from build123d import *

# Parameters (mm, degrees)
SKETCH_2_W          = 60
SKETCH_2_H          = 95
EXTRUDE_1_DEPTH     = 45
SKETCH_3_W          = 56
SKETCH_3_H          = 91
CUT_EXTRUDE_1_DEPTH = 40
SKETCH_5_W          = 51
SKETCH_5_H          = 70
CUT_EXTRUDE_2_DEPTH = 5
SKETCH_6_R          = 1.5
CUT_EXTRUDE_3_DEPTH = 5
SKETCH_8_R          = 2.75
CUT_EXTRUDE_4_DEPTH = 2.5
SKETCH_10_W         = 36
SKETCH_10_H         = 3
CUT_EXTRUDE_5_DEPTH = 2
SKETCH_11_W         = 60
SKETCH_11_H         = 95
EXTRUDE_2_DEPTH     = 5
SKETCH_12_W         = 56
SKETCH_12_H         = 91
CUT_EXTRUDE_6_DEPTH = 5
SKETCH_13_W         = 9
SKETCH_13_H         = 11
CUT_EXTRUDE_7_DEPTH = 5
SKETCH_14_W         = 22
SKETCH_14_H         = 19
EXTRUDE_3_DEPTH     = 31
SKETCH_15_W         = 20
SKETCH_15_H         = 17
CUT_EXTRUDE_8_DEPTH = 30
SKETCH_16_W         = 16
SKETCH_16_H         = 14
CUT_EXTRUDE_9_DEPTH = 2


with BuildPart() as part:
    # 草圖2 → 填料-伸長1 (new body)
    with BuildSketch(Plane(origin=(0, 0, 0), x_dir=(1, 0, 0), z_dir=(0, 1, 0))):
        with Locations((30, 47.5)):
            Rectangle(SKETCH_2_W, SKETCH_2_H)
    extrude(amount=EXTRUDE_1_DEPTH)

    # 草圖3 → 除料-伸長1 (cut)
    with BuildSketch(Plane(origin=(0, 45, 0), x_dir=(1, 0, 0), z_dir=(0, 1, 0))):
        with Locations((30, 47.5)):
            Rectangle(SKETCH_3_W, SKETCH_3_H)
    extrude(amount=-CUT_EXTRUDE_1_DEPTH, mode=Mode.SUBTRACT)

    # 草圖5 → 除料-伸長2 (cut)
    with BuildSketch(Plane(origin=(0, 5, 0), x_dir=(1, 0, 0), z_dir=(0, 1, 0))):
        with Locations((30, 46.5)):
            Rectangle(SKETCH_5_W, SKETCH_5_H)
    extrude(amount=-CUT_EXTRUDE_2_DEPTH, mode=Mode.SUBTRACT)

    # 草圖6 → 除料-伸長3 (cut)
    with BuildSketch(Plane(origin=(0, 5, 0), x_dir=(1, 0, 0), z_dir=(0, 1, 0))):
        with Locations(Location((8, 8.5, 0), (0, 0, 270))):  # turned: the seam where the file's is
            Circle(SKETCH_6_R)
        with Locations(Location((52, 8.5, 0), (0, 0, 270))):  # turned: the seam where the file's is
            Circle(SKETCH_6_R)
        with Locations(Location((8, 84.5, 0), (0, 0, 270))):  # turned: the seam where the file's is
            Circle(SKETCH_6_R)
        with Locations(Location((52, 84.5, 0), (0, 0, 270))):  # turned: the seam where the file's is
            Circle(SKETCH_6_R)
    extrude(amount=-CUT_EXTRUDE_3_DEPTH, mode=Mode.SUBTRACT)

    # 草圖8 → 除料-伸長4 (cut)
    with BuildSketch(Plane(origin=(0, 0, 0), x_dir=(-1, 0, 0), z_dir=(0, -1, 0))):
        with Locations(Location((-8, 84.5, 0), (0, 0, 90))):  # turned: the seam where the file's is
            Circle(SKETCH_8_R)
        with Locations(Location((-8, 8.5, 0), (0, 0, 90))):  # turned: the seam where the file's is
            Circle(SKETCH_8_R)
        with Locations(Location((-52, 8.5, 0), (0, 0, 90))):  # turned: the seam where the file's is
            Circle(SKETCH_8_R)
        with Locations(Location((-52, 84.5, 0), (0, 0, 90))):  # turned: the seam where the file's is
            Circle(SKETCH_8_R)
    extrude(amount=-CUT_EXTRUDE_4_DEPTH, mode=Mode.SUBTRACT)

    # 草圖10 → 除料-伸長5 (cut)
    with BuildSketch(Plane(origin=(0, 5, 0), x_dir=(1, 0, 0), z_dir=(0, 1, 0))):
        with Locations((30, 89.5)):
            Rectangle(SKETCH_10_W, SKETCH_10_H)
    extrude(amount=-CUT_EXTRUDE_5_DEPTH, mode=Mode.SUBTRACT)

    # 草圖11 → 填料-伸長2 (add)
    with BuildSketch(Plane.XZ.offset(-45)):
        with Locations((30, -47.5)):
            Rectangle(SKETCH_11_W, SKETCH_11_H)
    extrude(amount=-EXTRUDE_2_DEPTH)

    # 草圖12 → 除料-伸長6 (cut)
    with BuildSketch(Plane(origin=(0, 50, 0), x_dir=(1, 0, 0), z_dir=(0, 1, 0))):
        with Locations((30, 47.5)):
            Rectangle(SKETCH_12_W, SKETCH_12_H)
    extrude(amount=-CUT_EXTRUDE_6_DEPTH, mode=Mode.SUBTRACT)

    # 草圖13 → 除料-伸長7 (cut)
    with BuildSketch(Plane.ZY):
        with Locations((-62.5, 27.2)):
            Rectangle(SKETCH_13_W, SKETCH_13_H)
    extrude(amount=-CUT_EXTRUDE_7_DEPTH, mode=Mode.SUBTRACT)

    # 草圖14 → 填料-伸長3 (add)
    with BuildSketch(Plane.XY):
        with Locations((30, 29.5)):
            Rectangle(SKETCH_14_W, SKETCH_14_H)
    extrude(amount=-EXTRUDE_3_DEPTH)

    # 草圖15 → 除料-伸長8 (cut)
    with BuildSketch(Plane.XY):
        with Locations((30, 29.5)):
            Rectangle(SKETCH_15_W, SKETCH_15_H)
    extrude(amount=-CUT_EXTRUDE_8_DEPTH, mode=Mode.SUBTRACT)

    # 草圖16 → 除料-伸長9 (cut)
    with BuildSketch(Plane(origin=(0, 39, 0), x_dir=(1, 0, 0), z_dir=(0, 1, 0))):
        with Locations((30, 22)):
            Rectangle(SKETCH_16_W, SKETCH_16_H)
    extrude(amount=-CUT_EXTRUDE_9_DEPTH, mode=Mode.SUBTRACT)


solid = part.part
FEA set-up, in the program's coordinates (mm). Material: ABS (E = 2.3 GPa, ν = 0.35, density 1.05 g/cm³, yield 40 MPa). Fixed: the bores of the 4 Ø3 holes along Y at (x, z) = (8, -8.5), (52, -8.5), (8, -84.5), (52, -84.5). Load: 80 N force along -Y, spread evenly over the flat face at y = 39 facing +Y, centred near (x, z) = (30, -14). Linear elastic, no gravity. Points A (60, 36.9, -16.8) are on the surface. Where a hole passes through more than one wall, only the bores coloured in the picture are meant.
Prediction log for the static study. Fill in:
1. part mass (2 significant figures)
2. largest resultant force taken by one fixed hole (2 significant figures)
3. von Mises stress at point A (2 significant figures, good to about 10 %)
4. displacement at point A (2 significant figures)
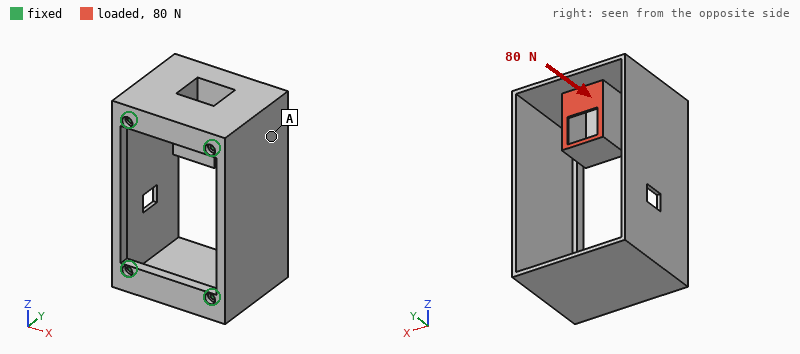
41 g
37 N
1.8 MPa
0.27 mm
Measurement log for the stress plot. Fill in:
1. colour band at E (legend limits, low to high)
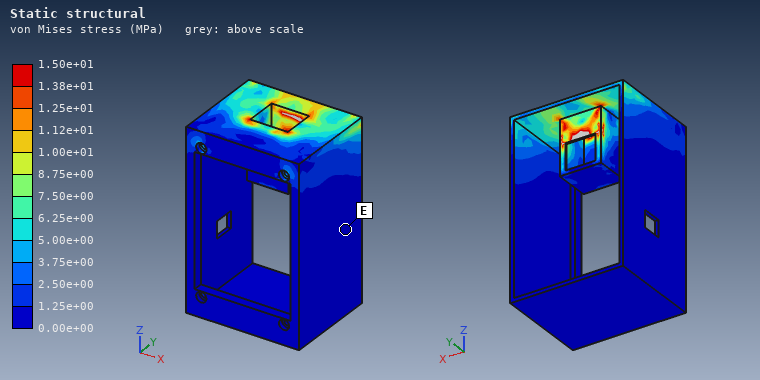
0.00e+00 to 1.25e+00 MPa
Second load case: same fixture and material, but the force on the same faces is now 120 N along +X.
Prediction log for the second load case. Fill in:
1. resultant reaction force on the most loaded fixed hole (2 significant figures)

120 N
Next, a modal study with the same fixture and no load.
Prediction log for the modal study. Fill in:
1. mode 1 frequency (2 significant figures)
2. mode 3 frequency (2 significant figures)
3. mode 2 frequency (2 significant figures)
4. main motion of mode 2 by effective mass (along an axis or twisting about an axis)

350 Hz
610 Hz
380 Hz
along X
